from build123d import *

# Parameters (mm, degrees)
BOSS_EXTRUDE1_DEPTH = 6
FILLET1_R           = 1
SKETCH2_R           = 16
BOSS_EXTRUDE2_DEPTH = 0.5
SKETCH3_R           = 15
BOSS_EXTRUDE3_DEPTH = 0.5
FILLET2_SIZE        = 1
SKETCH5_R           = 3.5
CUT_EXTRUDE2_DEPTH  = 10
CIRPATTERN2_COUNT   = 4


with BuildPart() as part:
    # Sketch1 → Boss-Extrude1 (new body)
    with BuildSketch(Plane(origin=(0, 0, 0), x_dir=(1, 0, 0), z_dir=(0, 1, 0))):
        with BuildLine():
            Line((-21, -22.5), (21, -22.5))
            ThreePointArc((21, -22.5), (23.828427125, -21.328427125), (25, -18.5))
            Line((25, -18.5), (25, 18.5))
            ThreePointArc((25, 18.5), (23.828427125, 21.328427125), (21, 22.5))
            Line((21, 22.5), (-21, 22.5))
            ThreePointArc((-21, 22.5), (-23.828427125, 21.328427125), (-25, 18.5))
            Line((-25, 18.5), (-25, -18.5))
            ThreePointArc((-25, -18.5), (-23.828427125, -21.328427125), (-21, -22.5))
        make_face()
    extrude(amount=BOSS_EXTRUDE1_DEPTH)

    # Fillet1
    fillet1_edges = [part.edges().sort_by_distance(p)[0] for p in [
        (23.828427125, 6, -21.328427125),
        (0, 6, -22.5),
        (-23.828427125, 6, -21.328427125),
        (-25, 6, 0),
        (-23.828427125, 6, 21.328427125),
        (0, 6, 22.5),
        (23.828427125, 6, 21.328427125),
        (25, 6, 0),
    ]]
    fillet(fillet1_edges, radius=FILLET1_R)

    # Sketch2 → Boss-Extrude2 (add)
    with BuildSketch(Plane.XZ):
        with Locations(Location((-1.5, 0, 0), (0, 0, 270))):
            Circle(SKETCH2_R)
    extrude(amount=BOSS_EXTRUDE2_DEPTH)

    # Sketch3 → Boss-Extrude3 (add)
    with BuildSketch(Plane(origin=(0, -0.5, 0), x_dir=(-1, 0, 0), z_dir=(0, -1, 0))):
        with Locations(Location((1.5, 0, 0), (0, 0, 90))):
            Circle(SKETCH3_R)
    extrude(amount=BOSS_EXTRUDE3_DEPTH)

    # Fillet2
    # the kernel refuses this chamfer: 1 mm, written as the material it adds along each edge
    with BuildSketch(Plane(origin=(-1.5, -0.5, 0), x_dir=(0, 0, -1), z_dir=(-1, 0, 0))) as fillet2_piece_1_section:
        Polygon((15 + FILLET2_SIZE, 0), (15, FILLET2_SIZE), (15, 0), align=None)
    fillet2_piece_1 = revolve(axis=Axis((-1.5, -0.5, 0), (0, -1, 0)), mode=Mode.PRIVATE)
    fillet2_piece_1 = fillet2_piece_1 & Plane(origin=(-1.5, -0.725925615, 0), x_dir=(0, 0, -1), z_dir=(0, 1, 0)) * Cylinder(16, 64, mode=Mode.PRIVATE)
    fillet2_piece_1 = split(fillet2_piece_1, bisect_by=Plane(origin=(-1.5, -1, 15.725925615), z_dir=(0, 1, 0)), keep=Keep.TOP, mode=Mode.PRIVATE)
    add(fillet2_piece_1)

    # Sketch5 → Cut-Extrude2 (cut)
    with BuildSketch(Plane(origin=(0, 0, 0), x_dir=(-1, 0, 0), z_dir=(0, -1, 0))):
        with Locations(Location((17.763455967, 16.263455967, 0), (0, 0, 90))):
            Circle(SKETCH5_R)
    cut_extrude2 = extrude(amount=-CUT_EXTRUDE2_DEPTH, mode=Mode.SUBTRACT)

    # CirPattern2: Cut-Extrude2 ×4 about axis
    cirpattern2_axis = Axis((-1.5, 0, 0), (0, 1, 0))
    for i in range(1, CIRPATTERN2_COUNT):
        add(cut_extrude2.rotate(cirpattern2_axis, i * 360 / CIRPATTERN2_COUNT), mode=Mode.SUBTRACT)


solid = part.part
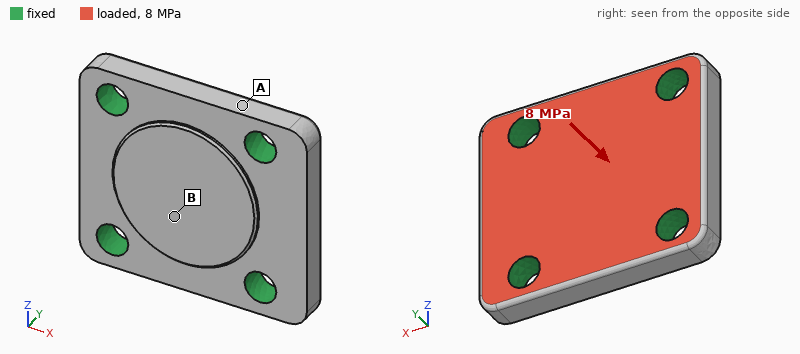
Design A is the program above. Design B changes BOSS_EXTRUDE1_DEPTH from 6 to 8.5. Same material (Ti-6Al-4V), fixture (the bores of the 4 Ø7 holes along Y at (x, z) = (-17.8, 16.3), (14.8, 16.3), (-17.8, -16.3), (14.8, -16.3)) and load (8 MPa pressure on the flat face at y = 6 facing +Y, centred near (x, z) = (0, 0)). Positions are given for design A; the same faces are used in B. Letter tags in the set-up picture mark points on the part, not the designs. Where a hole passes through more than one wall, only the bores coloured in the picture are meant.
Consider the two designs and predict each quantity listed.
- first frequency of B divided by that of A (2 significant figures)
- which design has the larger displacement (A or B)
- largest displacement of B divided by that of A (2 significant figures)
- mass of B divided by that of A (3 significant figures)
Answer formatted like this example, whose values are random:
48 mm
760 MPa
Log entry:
1.2
A
0.50
1.39
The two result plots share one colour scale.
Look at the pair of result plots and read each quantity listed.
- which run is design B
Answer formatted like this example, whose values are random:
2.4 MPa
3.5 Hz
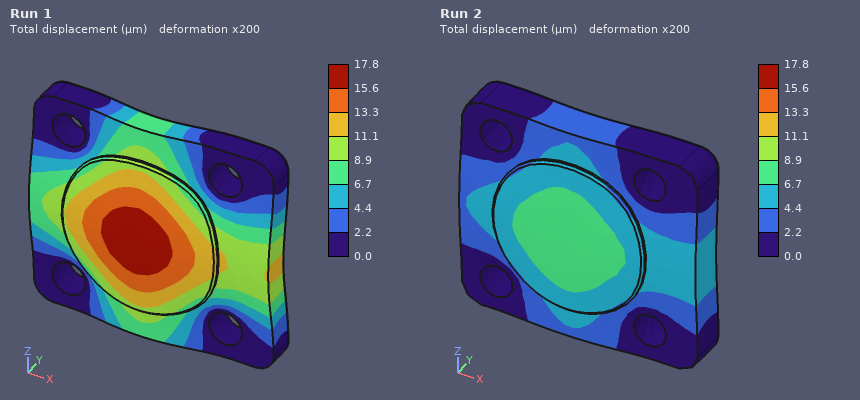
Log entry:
Run 2
